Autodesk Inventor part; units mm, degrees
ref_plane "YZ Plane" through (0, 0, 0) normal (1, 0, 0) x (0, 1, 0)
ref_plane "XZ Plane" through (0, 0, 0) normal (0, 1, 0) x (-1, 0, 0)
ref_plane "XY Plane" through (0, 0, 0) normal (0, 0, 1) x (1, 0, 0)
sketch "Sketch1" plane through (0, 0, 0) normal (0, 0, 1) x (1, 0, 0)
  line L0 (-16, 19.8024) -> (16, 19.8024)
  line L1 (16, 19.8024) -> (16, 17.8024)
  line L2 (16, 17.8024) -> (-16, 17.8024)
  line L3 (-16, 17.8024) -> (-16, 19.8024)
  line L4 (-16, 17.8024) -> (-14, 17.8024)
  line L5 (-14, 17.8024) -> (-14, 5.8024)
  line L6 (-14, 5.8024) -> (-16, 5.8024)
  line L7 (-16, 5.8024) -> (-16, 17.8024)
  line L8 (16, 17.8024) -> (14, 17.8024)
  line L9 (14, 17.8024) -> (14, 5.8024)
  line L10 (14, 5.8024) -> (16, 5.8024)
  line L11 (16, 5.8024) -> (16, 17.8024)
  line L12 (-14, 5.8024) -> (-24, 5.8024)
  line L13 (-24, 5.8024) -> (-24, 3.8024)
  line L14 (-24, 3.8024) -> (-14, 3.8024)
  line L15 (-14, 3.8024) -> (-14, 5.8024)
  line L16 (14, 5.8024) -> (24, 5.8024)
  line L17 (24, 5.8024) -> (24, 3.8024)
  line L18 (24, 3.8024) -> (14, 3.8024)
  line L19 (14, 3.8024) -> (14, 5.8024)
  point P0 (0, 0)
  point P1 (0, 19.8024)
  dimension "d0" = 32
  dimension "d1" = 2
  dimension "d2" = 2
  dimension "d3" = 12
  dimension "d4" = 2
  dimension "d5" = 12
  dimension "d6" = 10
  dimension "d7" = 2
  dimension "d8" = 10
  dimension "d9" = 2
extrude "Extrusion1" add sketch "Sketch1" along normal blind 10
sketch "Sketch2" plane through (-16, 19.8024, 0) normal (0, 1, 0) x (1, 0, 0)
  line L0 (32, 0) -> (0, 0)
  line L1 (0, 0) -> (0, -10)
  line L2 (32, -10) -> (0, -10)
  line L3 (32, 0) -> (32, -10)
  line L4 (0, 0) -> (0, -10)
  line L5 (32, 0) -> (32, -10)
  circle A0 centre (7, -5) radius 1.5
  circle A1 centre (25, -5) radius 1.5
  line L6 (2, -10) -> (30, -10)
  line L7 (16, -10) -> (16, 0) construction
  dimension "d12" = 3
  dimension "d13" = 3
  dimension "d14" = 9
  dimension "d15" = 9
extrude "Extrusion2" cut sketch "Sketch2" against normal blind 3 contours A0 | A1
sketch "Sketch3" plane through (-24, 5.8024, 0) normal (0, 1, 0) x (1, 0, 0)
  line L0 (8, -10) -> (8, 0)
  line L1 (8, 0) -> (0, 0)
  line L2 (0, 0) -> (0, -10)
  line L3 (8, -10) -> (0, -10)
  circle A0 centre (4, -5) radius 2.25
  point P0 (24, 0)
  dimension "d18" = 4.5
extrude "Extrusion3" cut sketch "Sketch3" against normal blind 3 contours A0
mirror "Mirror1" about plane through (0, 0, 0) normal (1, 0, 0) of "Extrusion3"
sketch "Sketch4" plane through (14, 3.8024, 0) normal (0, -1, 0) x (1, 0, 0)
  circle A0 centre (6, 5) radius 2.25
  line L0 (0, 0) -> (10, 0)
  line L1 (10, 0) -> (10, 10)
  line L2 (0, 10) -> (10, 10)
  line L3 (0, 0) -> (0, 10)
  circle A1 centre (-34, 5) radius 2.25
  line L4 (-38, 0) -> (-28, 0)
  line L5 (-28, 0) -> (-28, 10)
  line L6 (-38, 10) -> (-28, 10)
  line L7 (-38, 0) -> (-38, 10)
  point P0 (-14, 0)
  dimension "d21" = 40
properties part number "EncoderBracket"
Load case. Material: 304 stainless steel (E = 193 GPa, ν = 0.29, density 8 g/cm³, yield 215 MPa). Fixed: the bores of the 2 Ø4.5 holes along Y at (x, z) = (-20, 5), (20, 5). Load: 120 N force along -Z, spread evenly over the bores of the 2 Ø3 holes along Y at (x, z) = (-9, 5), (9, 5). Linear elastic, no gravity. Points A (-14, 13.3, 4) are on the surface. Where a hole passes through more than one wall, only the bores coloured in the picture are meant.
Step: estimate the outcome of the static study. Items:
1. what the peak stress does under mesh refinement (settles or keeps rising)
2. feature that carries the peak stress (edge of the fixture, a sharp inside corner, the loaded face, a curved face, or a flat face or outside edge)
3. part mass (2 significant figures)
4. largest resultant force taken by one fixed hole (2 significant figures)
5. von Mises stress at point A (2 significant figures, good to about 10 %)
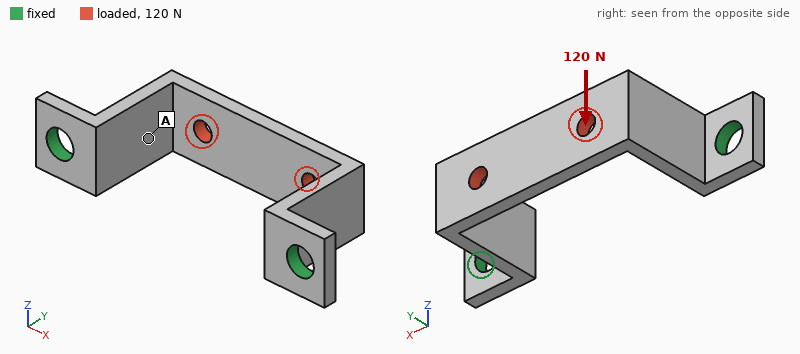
keeps rising
edge of the fixture
11 g
60 N
16 MPa
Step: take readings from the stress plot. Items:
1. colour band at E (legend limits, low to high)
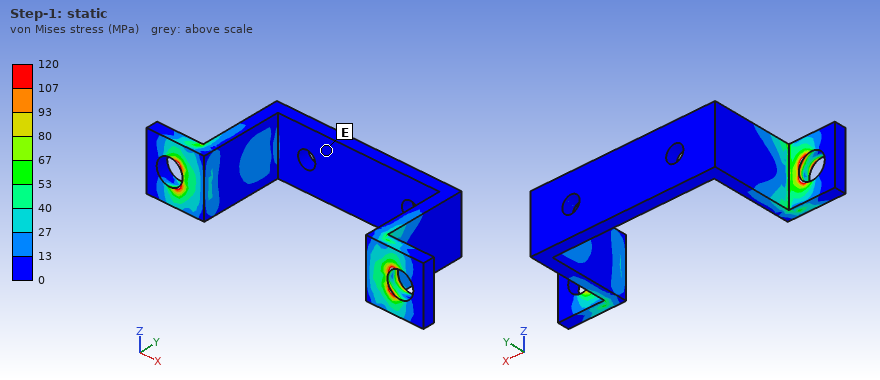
0 to 13 MPa
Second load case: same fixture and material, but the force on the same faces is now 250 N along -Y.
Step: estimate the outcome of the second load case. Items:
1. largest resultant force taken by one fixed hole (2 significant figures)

140 N
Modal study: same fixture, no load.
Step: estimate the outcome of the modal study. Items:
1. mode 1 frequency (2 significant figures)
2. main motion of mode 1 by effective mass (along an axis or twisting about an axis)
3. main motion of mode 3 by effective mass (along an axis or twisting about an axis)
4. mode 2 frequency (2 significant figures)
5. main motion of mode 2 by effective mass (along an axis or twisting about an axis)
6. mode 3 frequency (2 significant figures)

4400 Hz
along X
twisting about Y
5700 Hz
along Z
8500 Hz
